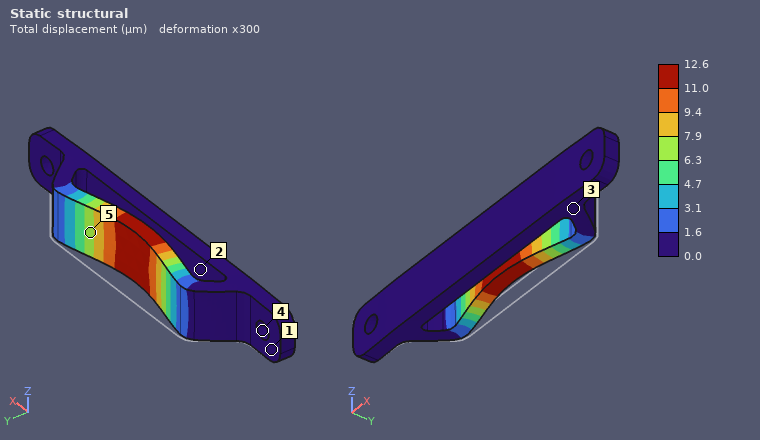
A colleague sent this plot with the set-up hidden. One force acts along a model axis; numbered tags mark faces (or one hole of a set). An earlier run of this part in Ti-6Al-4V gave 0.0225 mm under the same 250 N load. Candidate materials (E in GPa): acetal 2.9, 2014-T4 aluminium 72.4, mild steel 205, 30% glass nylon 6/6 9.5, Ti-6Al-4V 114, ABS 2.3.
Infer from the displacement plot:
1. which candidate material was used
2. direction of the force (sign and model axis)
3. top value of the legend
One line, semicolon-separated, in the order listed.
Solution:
mild steel; -Y; 12.6 µm
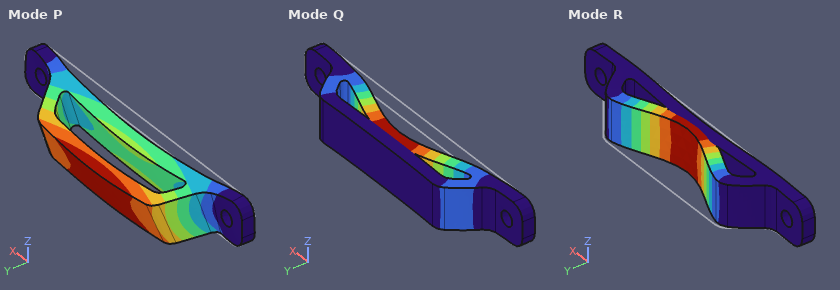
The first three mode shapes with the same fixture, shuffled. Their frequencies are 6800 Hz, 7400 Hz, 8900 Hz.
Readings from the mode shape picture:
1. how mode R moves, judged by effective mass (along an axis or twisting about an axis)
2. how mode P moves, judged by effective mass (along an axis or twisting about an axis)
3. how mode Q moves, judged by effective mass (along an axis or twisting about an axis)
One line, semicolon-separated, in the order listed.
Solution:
along Y; along Z; along Y
